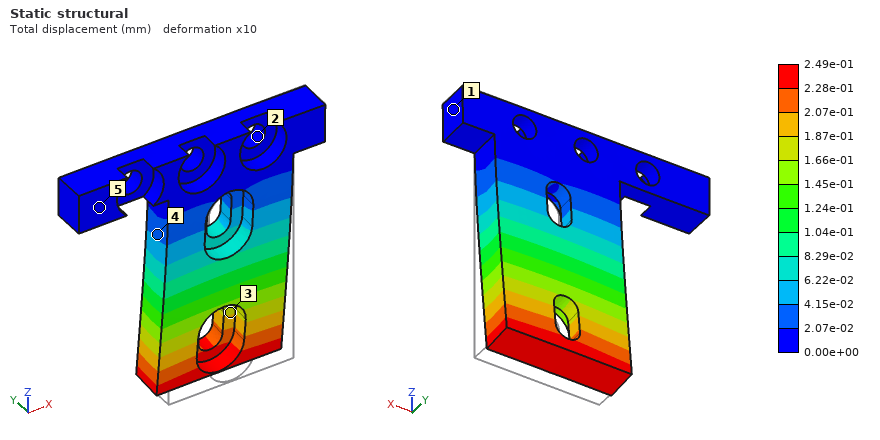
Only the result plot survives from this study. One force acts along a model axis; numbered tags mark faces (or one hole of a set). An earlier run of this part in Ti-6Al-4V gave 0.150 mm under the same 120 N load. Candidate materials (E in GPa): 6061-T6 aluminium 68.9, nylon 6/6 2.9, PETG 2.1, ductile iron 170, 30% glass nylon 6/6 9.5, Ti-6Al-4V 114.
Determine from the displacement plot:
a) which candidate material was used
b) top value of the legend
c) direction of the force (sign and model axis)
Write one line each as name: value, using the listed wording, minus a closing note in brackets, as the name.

which candidate material was used: 6061-T6 aluminium
top value of the legend: 2.49e-01 mm
direction of the force: +Y
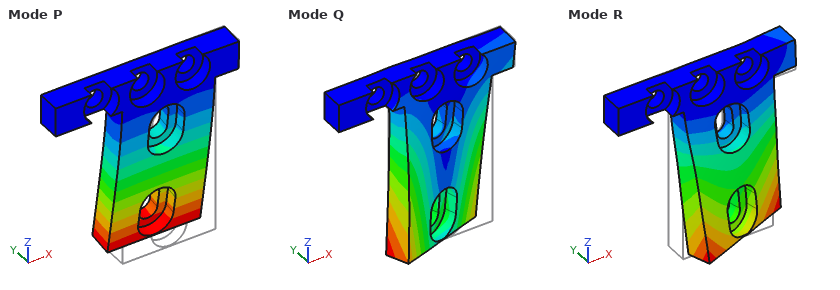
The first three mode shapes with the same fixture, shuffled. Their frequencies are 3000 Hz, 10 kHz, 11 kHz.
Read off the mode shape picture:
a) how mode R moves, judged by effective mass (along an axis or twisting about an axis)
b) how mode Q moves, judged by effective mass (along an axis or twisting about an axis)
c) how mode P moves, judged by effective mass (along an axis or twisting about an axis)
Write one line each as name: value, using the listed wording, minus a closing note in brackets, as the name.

how mode R moves, judged by effective mass: along X
how mode Q moves, judged by effective mass: along X
how mode P moves, judged by effective mass: along Y
